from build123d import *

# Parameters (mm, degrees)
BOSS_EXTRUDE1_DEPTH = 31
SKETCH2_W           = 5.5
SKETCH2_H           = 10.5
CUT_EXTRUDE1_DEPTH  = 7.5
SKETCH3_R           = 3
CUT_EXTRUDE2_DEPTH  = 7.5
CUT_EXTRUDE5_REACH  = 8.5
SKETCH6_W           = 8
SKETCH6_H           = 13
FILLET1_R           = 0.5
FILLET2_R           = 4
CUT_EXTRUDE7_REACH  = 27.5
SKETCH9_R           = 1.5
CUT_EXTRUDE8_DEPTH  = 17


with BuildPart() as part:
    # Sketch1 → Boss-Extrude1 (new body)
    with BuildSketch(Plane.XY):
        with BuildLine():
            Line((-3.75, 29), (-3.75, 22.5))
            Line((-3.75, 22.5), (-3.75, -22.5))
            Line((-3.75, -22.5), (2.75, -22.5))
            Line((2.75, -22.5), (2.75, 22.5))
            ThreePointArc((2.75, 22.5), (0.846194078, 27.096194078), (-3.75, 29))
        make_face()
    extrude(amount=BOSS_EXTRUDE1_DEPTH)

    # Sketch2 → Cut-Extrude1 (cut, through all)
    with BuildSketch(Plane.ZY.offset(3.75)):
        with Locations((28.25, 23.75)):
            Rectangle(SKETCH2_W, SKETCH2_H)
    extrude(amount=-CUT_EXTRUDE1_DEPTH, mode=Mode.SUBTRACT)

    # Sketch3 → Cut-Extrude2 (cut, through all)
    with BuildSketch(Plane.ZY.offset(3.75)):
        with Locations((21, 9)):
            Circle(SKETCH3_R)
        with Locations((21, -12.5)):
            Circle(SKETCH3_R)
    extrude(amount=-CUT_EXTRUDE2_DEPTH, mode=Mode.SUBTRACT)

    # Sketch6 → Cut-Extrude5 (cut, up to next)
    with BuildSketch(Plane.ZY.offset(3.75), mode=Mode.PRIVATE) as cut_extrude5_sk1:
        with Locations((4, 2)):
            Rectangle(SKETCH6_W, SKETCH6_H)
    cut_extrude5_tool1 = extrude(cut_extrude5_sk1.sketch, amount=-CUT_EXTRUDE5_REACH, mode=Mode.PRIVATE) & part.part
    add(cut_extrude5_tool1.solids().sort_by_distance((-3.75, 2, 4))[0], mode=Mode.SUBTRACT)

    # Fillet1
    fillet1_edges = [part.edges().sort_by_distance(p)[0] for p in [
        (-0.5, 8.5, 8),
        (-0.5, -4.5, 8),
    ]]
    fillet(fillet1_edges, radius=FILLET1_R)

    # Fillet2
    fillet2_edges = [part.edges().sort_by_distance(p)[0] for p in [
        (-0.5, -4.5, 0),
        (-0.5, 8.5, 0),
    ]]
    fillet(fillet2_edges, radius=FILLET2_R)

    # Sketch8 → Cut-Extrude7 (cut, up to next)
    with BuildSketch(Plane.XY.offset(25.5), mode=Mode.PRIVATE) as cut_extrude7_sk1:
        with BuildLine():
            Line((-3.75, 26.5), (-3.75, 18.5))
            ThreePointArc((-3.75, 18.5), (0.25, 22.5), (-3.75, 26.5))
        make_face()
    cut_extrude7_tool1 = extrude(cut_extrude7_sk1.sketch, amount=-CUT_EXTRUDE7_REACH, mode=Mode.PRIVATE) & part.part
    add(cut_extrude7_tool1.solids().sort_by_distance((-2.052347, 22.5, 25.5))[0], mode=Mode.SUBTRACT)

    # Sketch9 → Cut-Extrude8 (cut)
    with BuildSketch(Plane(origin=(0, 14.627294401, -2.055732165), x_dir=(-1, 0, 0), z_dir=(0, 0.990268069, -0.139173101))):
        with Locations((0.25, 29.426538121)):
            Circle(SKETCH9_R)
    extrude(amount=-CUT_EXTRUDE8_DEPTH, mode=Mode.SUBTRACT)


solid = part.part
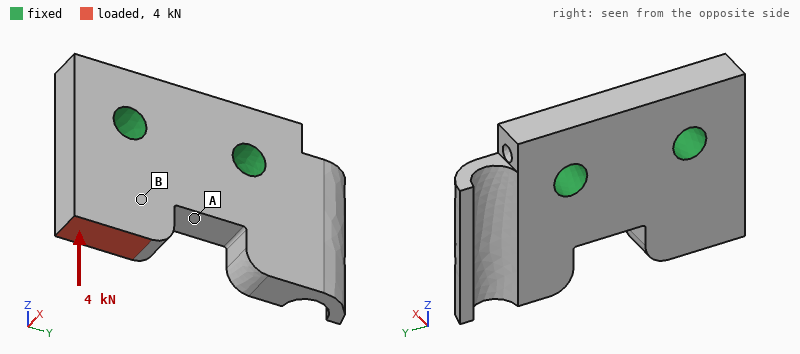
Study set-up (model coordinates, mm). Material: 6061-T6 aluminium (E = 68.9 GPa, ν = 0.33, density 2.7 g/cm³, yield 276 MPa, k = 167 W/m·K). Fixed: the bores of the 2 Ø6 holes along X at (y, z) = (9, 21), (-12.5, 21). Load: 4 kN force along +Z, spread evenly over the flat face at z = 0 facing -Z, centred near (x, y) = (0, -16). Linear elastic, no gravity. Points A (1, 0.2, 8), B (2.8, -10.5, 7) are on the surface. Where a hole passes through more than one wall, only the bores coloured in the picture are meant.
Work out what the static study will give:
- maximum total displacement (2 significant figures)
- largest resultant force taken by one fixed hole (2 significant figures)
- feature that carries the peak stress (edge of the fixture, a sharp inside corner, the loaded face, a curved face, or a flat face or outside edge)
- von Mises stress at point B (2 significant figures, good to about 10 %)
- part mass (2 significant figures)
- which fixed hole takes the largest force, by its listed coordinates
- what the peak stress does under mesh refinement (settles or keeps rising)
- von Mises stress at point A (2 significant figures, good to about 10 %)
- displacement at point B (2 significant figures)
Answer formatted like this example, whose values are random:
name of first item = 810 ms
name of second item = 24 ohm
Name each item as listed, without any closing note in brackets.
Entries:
maximum total displacement = 24 µm
largest resultant force taken by one fixed hole = 4.2 kN
feature that carries the peak stress = edge of the fixture
von Mises stress at point B = 38 MPa
part mass = 21 g
which fixed hole takes the largest force, by its listed coordinates = (-12.5, 21)
what the peak stress does under mesh refinement = keeps rising
von Mises stress at point A = 12 MPa
displacement at point B = 7.9 µm
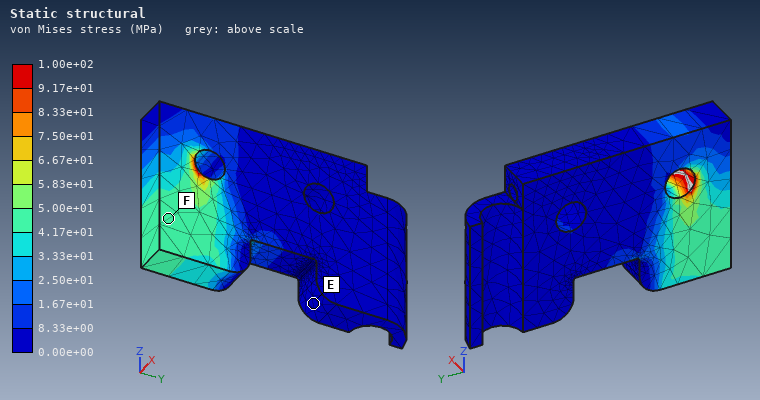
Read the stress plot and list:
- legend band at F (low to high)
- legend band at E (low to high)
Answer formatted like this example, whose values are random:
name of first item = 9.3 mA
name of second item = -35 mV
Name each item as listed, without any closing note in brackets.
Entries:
legend band at F = 4.17e+01 to 5.00e+01 MPa
legend band at E = 0.00e+00 to 8.33e+00 MPa
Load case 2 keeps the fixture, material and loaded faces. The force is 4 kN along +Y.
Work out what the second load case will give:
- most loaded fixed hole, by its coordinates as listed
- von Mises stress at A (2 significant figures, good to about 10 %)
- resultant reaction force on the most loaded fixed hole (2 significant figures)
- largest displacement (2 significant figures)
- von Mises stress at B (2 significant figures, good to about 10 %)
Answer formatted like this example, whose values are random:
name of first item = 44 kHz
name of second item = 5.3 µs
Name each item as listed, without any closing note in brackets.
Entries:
most loaded fixed hole, by its coordinates as listed = (9, 21)
von Mises stress at A = 56 MPa
resultant reaction force on the most loaded fixed hole = 3.8 kN
largest displacement = 73 µm
von Mises stress at B = 90 MPa
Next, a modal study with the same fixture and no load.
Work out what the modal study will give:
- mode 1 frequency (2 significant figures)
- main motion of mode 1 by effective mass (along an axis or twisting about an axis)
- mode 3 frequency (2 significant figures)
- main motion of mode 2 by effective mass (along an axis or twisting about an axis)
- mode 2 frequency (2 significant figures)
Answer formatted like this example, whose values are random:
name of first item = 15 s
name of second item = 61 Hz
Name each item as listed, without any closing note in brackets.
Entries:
mode 1 frequency = 10 kHz
main motion of mode 1 by effective mass = along X
mode 3 frequency = 16 kHz
main motion of mode 2 by effective mass = along X
mode 2 frequency = 14 kHz
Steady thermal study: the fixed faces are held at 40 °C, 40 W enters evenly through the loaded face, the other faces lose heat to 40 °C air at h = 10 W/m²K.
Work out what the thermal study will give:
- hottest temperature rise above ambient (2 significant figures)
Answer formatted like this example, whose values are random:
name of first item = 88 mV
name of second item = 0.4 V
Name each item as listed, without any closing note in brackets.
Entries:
hottest temperature rise above ambient = 42 K
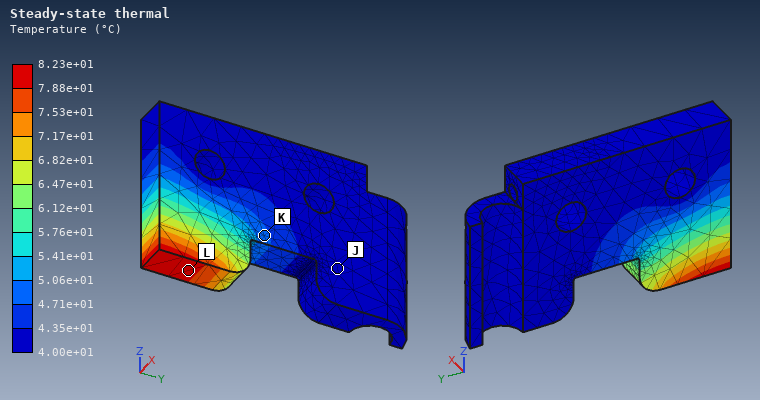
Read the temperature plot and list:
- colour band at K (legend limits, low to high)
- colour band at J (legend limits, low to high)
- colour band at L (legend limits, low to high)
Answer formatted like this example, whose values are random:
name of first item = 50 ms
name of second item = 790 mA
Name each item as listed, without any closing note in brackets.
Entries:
colour band at K = 4.71e+01 to 5.06e+01 °C
colour band at J = 4.00e+01 to 4.35e+01 °C
colour band at L = 7.88e+01 to 8.23e+01 °C
